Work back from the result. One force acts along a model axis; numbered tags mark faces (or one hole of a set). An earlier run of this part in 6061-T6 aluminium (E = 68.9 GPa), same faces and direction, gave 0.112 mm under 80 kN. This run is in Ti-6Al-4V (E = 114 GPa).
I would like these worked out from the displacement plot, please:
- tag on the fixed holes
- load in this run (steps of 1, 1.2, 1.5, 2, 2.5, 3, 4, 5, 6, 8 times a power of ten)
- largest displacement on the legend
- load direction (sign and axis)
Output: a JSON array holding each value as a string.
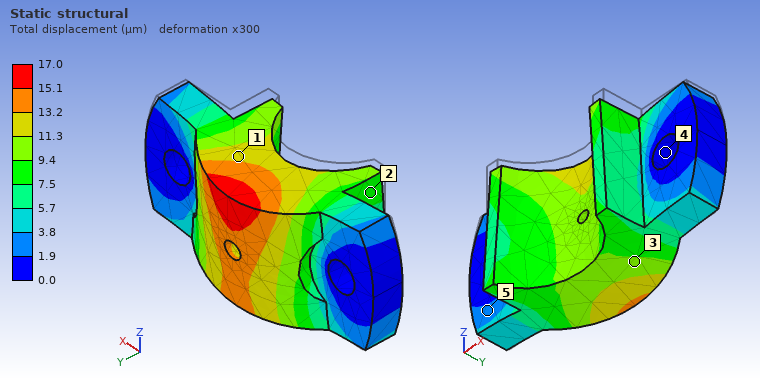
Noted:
["4", "20 kN", "17.0 µm", "-Z"]
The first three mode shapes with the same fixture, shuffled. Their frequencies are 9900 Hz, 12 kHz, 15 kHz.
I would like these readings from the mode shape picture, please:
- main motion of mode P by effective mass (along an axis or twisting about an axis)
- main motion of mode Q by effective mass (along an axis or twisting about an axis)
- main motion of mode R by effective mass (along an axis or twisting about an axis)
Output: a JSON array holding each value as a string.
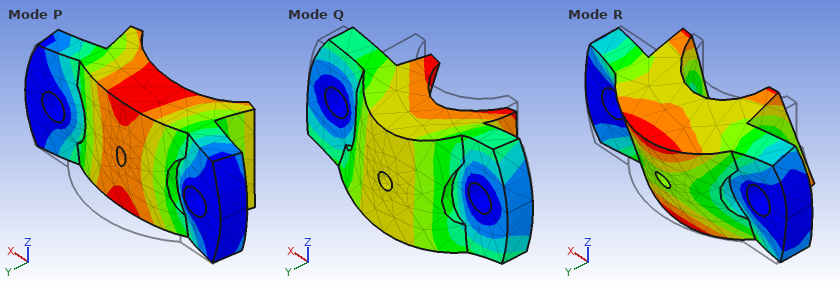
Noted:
["along Y", "along Z", "twisting about X"]
